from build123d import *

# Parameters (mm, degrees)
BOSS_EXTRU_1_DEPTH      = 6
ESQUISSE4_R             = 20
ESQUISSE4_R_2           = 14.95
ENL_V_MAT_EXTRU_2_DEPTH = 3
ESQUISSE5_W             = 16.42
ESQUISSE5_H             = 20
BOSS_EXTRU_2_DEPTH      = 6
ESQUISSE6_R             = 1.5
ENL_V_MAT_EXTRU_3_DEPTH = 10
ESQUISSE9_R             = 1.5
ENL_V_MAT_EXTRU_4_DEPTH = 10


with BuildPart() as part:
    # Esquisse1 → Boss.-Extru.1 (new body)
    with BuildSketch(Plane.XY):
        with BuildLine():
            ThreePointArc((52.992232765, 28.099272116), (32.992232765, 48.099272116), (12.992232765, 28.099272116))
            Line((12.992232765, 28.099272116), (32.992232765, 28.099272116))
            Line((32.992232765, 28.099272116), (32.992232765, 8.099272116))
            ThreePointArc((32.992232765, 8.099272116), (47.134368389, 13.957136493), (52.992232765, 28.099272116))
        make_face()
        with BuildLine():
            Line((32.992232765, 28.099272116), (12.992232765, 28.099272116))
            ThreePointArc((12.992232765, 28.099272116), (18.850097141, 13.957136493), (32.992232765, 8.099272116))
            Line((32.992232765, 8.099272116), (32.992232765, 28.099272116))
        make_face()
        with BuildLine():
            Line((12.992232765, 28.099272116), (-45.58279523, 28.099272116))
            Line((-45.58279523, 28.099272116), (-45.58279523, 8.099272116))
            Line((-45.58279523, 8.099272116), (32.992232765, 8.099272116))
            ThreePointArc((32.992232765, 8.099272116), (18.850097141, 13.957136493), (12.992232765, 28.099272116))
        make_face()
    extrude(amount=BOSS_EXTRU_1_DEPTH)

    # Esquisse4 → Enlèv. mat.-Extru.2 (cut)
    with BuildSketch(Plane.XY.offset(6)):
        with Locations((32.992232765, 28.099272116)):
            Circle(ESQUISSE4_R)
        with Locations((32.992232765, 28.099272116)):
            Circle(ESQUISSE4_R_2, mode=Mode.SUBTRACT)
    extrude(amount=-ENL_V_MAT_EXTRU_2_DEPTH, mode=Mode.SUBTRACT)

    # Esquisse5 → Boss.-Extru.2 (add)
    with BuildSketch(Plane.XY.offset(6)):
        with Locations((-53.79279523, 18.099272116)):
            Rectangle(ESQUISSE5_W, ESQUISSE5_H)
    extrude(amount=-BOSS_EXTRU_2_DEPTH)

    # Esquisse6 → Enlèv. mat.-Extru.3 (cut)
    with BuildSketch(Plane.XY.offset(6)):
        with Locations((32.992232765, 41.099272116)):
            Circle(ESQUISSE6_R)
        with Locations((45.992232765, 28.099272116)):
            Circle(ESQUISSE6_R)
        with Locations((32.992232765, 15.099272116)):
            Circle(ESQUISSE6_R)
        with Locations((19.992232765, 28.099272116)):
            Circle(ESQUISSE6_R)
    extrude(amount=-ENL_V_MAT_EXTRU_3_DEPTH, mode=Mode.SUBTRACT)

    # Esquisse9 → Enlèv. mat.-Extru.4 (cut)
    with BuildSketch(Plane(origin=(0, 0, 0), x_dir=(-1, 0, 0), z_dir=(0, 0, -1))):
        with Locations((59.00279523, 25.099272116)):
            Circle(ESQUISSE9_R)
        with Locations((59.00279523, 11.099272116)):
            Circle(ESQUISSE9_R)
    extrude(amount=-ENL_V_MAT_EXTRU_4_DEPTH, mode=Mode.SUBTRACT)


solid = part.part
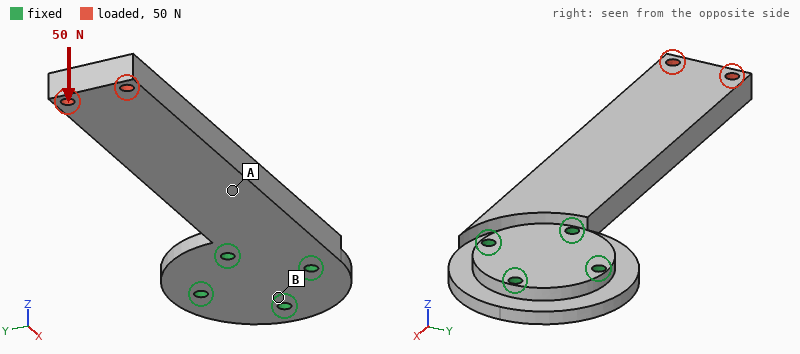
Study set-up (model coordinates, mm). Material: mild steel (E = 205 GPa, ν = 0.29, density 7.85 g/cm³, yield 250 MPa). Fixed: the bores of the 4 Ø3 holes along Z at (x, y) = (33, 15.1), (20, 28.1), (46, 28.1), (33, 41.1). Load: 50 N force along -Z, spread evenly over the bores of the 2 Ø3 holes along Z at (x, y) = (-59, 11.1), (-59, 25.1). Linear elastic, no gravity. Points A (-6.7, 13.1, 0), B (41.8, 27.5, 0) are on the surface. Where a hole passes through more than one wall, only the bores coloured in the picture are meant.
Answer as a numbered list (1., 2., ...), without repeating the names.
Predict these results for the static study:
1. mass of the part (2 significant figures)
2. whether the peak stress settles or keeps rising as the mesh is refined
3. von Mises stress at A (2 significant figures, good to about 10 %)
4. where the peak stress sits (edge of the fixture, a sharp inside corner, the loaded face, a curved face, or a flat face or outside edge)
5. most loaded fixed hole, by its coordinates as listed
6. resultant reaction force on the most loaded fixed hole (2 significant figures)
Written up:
1. 120 g
2. keeps rising
3. 22 MPa
4. edge of the fixture
5. (20, 28.1)
6. 210 N
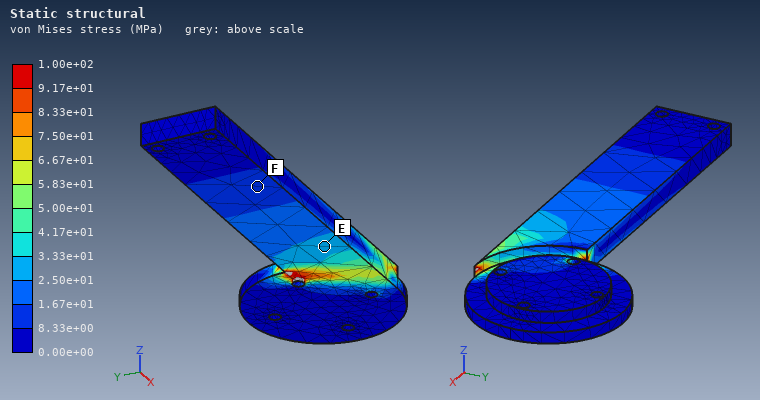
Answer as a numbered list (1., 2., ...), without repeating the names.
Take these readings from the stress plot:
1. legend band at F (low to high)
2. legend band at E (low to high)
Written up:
1. 8.33e+00 to 1.67e+01 MPa
2. 2.50e+01 to 3.33e+01 MPa
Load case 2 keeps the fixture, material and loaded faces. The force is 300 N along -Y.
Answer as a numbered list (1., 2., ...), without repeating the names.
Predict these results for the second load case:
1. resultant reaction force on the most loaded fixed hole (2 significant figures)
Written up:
1. 1.2 kN
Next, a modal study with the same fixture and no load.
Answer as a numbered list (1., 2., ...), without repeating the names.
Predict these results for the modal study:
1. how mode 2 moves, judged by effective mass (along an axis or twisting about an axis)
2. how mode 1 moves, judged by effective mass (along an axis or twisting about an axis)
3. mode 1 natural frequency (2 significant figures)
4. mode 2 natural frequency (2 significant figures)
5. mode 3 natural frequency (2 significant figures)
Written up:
1. along Y
2. along Z
3. 470 Hz
4. 2000 Hz
5. 3300 Hz
